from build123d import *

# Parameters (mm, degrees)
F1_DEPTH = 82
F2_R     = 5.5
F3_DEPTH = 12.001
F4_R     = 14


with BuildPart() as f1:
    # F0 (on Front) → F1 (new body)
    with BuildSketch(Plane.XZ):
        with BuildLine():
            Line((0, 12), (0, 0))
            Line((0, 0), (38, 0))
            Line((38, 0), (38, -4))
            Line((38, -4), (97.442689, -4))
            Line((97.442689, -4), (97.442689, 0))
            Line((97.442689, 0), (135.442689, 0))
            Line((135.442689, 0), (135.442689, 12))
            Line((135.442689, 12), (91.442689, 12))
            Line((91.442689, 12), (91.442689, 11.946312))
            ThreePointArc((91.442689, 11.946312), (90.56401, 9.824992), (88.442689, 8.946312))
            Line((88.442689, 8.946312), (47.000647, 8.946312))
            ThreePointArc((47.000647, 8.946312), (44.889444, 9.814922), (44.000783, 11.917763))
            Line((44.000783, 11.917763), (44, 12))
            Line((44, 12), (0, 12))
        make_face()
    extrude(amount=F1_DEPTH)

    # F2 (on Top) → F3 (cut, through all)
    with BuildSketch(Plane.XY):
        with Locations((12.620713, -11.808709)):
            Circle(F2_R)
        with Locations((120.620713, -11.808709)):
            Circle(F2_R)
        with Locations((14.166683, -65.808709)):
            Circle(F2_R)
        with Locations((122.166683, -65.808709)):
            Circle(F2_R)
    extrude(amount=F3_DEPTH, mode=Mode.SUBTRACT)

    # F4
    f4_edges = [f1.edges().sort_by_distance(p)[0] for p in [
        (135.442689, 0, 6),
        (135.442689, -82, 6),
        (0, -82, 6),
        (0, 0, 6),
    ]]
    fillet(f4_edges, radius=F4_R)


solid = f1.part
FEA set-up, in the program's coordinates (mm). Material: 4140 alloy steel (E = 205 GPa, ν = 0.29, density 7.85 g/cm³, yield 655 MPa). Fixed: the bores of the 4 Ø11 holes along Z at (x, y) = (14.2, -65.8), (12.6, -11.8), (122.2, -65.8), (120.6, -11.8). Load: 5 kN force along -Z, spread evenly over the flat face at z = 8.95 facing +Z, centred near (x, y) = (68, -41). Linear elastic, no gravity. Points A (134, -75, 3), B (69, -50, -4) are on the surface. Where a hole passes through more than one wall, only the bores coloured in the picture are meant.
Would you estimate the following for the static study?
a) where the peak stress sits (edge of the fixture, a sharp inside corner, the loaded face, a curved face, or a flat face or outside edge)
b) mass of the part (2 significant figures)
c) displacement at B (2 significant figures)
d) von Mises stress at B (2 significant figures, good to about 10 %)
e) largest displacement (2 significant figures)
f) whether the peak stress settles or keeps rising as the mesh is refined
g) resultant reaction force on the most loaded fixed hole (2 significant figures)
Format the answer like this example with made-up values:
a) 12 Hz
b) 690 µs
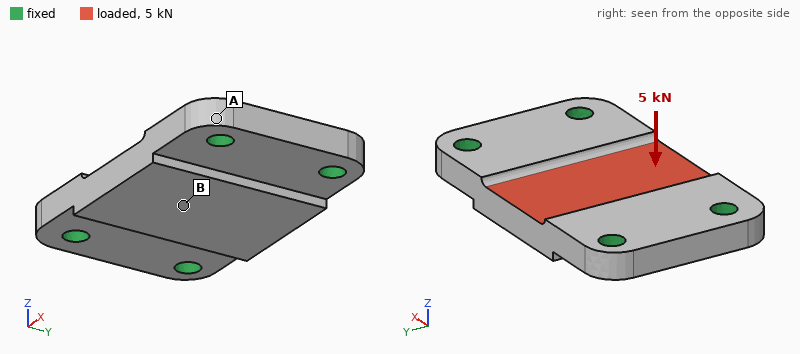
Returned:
a) edge of the fixture
b) 1.1 kg
c) 10 µm
d) 18 MPa
e) 11 µm
f) keeps rising
g) 2.1 kN
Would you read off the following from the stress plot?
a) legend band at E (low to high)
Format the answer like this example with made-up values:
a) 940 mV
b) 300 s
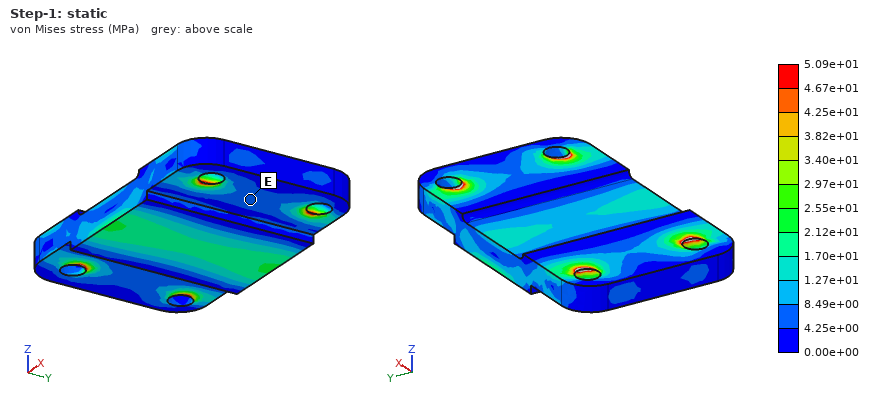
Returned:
a) 4.25e+00 to 8.49e+00 MPa
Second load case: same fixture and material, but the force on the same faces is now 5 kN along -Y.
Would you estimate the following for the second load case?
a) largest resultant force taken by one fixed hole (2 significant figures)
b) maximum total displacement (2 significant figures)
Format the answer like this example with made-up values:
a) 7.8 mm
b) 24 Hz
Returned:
a) 1.5 kN
b) 3.0 µm
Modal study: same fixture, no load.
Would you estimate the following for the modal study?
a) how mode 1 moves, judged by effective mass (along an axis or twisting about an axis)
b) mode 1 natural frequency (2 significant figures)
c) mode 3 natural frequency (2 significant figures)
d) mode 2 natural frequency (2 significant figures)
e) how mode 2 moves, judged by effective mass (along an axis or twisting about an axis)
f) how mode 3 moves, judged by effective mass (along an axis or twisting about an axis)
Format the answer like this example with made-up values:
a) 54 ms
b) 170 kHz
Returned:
a) along Z
b) 5400 Hz
c) 12 kHz
d) 7000 Hz
e) twisting about X
f) along Y
